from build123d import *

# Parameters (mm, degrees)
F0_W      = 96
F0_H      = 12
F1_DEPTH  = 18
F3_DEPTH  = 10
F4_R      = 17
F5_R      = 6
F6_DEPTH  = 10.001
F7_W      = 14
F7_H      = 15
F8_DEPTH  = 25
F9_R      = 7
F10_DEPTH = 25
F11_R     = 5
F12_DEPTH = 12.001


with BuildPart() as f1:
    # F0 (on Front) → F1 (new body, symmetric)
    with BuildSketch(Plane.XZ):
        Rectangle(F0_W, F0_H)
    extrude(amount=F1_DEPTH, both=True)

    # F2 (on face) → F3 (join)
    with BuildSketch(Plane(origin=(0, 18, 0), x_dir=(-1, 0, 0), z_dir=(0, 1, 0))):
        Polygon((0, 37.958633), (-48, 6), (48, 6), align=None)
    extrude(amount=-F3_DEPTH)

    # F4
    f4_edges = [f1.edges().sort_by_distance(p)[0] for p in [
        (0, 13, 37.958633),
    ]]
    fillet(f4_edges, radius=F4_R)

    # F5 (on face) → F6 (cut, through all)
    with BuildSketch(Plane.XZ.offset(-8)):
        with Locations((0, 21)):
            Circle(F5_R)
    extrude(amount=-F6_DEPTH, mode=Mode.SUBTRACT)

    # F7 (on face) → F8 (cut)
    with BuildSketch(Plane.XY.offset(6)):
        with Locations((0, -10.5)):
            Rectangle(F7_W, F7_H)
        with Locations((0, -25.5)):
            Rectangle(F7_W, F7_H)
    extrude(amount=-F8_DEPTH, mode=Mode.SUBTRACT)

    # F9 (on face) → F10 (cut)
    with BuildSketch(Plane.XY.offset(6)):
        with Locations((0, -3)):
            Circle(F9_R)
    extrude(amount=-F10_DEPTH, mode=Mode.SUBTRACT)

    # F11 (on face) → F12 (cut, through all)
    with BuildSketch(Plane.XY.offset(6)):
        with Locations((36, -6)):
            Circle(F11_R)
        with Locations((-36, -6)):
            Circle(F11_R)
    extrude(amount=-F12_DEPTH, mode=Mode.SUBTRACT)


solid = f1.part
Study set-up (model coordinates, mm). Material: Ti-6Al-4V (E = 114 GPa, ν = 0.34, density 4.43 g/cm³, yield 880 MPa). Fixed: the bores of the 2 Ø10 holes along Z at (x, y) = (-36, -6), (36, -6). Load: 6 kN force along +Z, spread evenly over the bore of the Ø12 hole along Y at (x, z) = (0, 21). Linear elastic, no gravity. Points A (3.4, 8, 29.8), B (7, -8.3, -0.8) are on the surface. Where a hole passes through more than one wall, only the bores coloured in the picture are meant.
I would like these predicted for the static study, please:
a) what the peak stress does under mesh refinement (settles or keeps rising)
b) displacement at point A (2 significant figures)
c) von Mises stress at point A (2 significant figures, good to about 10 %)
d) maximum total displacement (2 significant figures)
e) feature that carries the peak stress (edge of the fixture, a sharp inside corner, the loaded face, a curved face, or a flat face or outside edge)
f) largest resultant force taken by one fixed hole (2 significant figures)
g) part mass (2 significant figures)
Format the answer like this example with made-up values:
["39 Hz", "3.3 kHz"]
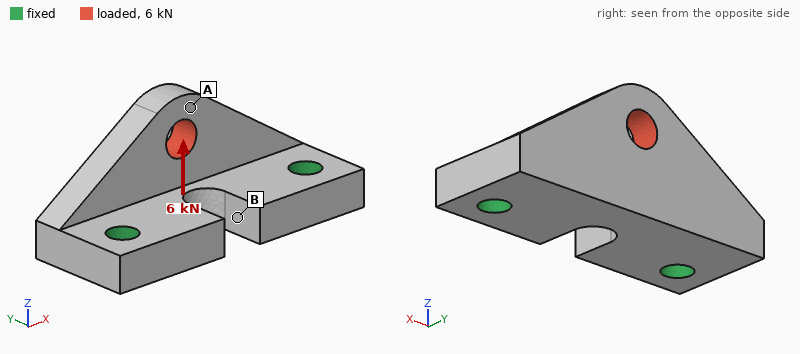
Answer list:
["keeps rising", "39 µm", "33 MPa", "50 µm", "edge of the fixture", "3.1 kN", "220 g"]
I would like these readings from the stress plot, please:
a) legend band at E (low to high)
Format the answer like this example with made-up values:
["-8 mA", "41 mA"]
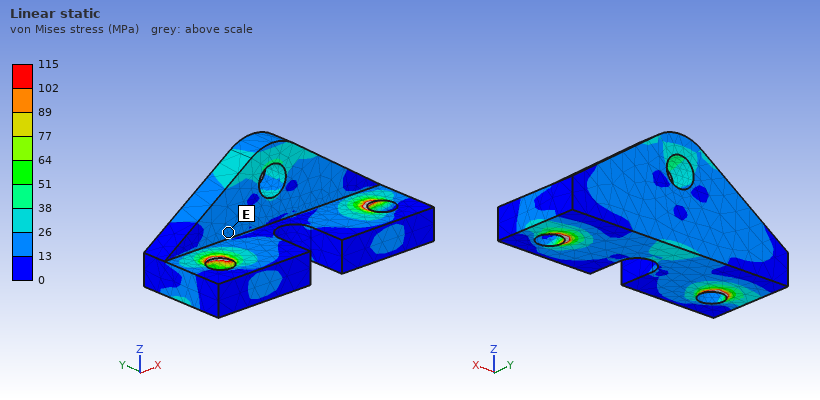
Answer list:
["13 to 26 MPa"]
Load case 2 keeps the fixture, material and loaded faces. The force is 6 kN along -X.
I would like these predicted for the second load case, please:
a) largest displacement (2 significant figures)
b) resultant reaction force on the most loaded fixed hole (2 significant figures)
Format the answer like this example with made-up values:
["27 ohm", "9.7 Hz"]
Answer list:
["17 µm", "3.6 kN"]
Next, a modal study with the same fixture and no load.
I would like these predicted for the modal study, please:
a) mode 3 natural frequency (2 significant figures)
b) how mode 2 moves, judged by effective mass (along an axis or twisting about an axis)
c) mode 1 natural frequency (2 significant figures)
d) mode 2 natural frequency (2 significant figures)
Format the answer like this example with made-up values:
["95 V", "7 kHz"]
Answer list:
["12 kHz", "along Z", "5900 Hz", "11 kHz"]
